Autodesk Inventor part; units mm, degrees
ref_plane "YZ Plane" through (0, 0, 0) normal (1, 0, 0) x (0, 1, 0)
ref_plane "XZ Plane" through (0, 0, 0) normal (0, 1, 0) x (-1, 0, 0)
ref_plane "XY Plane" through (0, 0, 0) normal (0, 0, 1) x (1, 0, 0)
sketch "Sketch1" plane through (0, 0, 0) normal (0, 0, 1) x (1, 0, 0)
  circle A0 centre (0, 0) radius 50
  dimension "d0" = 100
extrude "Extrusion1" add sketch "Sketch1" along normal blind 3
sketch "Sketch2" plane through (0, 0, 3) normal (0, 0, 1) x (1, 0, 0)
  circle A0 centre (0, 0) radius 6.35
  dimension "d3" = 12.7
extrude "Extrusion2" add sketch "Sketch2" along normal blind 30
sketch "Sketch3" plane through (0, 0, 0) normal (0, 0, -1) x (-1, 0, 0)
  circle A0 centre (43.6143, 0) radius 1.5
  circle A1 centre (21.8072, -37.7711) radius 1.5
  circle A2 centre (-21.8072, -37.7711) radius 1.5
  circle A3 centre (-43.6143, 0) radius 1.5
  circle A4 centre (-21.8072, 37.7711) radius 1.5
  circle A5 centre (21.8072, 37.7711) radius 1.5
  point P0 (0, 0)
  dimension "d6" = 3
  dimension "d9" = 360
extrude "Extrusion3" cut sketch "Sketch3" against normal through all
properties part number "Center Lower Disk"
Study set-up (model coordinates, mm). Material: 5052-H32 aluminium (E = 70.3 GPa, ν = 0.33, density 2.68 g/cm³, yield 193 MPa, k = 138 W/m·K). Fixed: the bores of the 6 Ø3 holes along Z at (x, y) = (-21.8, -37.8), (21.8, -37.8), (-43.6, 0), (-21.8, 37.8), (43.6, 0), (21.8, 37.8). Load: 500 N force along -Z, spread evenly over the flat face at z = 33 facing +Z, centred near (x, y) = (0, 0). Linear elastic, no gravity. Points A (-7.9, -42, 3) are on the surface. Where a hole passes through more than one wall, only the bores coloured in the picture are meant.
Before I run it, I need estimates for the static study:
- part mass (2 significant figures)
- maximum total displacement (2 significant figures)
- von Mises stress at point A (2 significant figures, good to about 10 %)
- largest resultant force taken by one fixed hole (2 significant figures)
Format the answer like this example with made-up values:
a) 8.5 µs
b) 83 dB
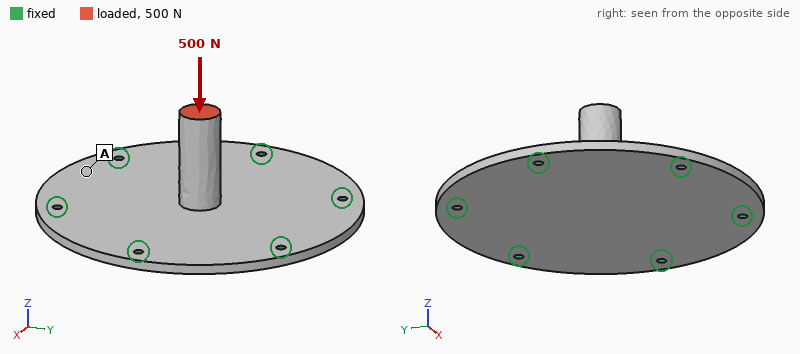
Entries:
a) 73 g
b) 0.11 mm
c) 9.3 MPa
d) 85 N
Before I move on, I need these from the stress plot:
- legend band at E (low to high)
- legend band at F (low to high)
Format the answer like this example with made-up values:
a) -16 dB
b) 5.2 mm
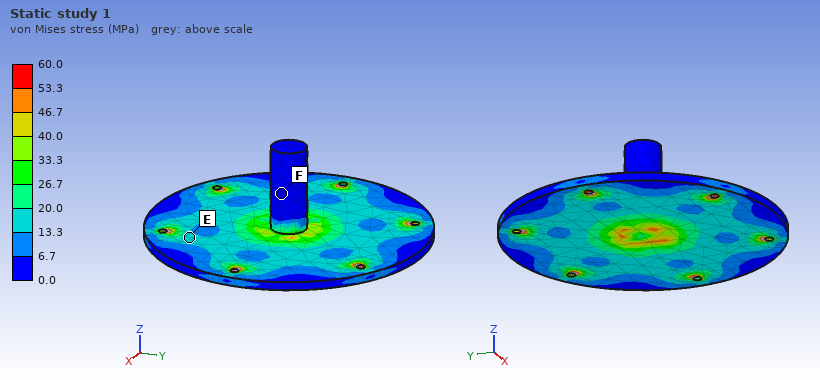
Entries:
a) 13.3 to 20.0 MPa
b) 0.0 to 6.7 MPa
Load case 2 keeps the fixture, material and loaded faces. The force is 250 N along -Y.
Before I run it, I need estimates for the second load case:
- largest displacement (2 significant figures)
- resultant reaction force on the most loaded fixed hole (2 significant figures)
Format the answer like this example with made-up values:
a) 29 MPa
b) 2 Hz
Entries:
a) 0.18 mm
b) 88 N
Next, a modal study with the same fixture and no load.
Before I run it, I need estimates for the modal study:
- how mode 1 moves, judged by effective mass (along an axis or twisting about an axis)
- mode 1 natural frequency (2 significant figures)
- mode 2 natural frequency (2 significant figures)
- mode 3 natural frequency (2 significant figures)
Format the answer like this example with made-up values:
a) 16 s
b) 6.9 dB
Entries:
a) along Z
b) 2400 Hz
c) 3000 Hz
d) 3000 Hz
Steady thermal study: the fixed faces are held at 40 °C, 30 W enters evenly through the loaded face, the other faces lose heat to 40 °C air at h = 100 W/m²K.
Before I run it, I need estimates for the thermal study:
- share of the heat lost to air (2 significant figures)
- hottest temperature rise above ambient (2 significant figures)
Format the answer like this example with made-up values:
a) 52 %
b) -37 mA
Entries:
a) 43 %
b) 67 K
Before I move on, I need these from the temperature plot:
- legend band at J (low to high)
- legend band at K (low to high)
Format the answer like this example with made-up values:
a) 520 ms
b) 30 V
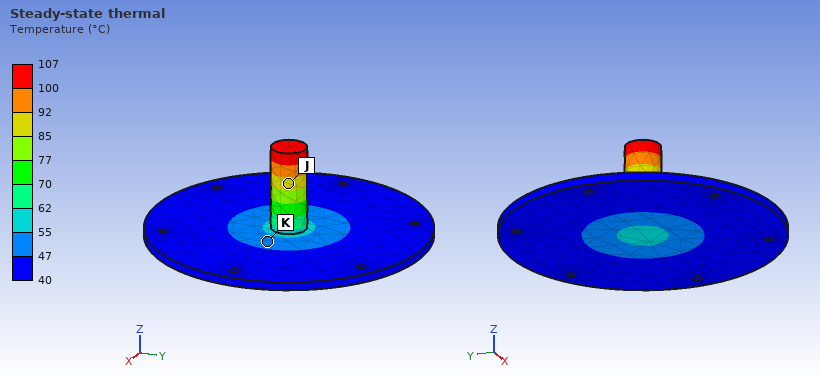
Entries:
a) 85 to 92 °C
b) 47 to 55 °C
